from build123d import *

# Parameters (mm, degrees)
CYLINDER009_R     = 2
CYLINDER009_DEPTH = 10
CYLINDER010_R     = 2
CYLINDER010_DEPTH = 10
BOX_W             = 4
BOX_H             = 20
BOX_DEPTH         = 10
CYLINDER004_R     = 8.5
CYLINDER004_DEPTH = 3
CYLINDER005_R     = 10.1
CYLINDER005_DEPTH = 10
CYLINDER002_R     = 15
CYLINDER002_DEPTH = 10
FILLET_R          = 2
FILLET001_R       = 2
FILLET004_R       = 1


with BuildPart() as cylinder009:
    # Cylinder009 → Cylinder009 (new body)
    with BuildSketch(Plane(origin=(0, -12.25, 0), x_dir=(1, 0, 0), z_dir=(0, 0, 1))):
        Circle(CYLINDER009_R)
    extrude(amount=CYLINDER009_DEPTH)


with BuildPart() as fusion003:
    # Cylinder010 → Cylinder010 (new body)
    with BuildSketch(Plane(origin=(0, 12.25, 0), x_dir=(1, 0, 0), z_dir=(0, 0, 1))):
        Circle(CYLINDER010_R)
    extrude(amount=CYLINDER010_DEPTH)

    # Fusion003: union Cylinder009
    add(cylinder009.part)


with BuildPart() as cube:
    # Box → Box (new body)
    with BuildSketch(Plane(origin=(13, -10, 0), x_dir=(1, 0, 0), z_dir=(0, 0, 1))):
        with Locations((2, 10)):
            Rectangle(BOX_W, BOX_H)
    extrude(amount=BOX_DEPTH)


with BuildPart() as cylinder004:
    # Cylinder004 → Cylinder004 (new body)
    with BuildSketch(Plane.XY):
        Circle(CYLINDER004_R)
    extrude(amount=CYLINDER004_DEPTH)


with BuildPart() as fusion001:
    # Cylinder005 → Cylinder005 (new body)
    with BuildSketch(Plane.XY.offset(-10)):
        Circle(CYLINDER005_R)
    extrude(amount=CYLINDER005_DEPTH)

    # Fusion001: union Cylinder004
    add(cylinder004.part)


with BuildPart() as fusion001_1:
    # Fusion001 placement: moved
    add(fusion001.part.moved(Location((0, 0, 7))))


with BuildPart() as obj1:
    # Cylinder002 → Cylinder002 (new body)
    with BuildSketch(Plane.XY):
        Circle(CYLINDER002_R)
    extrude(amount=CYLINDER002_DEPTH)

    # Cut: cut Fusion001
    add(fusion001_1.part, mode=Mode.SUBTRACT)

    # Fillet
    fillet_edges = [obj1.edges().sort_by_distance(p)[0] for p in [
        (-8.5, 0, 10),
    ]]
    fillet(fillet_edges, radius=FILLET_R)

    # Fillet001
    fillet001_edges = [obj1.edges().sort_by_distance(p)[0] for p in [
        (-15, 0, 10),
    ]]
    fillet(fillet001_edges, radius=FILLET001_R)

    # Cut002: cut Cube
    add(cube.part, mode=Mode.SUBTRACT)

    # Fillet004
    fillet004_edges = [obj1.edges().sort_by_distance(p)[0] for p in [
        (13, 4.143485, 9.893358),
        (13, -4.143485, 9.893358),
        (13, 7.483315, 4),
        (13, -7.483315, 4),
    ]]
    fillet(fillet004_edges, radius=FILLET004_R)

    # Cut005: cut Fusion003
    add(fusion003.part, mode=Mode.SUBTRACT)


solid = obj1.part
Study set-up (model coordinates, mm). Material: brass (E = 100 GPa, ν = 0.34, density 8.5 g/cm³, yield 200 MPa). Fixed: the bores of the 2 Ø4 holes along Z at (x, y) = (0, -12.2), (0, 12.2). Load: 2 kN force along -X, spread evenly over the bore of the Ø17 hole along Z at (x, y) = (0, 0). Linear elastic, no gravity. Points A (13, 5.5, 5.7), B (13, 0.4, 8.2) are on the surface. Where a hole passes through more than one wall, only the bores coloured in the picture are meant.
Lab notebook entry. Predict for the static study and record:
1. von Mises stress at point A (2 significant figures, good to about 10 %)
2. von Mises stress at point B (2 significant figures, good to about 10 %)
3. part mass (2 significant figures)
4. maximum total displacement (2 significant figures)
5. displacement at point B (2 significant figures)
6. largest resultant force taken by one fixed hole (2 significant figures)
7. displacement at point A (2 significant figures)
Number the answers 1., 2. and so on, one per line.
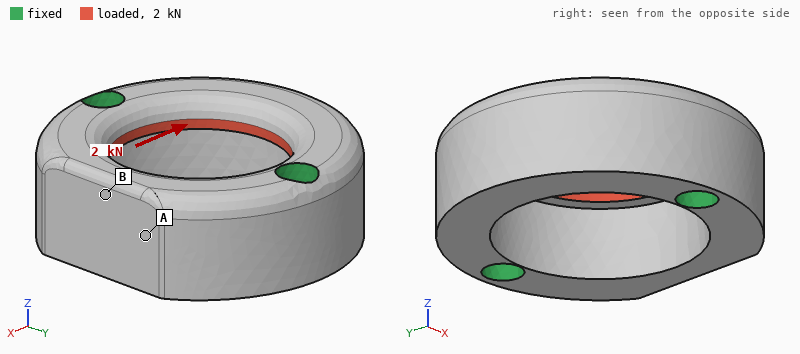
1. 9.6 MPa
2. 30 MPa
3. 30 g
4. 4.9 µm
5. 4.2 µm
6. 1.0 kN
7. 2.5 µm
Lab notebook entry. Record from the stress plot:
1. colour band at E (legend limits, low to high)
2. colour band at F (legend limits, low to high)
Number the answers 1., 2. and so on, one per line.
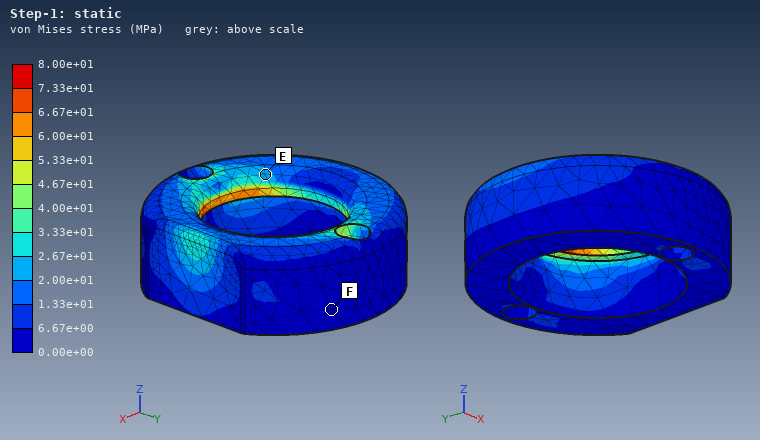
1. 2.00e+01 to 2.67e+01 MPa
2. 0.00e+00 to 6.67e+00 MPa
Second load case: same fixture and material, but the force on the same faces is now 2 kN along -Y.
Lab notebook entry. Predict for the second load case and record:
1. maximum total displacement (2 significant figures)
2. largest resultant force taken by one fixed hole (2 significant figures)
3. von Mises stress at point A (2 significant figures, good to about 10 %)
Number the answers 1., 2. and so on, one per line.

1. 5.2 µm
2. 1.0 kN
3. 12 MPa
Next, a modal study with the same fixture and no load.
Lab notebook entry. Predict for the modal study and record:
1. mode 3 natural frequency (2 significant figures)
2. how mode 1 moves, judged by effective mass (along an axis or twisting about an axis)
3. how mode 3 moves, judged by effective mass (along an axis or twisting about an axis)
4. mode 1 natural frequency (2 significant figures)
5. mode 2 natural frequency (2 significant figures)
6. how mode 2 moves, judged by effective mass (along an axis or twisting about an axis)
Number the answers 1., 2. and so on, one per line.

1. 22 kHz
2. along Z
3. along Y
4. 16 kHz
5. 19 kHz
6. along Z
